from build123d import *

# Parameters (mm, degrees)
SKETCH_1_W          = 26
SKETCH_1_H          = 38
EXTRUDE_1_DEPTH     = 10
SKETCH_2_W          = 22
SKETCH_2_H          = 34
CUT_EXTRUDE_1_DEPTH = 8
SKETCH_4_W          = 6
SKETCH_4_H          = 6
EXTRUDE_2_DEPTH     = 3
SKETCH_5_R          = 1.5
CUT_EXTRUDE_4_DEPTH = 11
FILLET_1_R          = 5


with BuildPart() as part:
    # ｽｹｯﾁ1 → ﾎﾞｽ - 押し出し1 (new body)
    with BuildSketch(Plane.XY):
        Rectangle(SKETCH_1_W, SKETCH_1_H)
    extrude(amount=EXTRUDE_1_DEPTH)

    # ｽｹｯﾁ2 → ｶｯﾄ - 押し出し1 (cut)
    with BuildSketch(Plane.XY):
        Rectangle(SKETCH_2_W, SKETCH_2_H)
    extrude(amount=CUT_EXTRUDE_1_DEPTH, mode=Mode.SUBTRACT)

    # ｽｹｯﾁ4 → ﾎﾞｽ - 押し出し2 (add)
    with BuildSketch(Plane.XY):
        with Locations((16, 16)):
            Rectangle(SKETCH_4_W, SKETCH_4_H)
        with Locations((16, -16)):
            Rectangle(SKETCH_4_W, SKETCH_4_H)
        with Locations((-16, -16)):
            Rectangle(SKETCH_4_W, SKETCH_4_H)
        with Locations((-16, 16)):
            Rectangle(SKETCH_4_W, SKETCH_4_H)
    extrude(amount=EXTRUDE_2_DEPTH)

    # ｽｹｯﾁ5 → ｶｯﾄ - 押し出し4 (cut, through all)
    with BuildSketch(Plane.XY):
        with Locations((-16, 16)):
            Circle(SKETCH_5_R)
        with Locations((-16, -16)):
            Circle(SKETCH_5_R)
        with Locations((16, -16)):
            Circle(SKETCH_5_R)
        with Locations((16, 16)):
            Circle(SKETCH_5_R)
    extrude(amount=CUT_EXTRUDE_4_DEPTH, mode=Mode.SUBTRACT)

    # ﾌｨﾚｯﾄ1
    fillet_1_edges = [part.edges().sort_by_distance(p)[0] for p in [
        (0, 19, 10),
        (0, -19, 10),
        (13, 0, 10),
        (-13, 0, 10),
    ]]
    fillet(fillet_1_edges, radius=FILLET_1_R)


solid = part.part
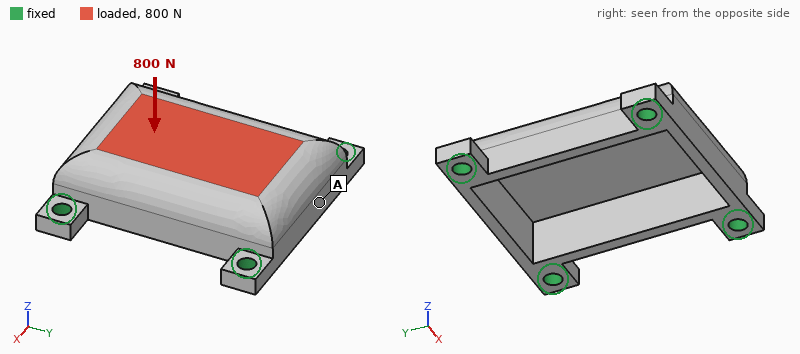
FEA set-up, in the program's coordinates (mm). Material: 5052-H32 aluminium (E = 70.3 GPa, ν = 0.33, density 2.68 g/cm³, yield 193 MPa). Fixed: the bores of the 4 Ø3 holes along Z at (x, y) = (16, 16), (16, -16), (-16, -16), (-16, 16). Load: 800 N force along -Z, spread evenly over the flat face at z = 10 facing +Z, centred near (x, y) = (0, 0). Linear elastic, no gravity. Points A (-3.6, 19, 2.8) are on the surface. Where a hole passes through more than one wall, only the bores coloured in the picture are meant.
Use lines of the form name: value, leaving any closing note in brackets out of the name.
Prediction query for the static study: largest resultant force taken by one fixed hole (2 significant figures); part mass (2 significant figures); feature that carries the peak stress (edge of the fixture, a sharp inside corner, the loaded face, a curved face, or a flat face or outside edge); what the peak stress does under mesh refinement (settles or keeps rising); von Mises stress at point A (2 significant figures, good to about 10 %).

largest resultant force taken by one fixed hole: 260 N
part mass: 9.7 g
feature that carries the peak stress: edge of the fixture
what the peak stress does under mesh refinement: keeps rising
von Mises stress at point A: 12 MPa
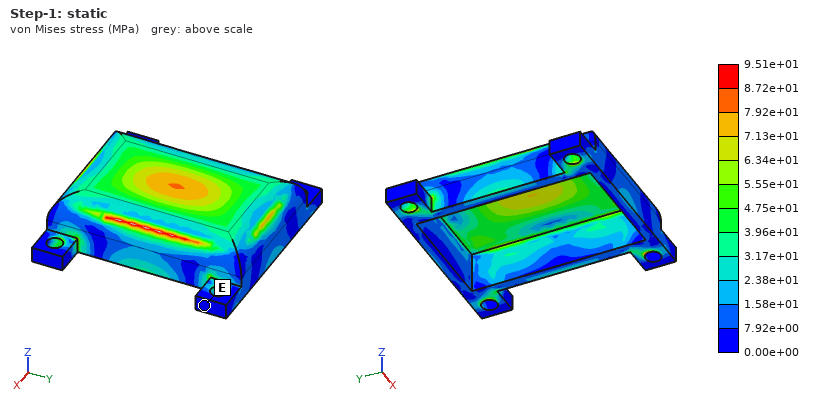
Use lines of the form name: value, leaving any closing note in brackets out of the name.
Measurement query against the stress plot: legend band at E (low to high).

legend band at E: 0.00e+00 to 7.92e+00 MPa
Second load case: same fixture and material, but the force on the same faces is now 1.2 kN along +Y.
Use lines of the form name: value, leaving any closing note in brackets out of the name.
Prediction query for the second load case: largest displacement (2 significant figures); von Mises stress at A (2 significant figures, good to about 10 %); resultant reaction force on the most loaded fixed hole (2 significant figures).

largest displacement: 12 µm
von Mises stress at A: 8.3 MPa
resultant reaction force on the most loaded fixed hole: 330 N
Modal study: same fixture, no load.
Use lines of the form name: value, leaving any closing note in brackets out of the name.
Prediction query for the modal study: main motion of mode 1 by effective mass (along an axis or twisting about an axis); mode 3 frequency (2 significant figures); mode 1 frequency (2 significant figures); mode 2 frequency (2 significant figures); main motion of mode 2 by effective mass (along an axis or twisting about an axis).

main motion of mode 1 by effective mass: along Z
mode 3 frequency: 19 kHz
mode 1 frequency: 13 kHz
mode 2 frequency: 17 kHz
main motion of mode 2 by effective mass: along X
